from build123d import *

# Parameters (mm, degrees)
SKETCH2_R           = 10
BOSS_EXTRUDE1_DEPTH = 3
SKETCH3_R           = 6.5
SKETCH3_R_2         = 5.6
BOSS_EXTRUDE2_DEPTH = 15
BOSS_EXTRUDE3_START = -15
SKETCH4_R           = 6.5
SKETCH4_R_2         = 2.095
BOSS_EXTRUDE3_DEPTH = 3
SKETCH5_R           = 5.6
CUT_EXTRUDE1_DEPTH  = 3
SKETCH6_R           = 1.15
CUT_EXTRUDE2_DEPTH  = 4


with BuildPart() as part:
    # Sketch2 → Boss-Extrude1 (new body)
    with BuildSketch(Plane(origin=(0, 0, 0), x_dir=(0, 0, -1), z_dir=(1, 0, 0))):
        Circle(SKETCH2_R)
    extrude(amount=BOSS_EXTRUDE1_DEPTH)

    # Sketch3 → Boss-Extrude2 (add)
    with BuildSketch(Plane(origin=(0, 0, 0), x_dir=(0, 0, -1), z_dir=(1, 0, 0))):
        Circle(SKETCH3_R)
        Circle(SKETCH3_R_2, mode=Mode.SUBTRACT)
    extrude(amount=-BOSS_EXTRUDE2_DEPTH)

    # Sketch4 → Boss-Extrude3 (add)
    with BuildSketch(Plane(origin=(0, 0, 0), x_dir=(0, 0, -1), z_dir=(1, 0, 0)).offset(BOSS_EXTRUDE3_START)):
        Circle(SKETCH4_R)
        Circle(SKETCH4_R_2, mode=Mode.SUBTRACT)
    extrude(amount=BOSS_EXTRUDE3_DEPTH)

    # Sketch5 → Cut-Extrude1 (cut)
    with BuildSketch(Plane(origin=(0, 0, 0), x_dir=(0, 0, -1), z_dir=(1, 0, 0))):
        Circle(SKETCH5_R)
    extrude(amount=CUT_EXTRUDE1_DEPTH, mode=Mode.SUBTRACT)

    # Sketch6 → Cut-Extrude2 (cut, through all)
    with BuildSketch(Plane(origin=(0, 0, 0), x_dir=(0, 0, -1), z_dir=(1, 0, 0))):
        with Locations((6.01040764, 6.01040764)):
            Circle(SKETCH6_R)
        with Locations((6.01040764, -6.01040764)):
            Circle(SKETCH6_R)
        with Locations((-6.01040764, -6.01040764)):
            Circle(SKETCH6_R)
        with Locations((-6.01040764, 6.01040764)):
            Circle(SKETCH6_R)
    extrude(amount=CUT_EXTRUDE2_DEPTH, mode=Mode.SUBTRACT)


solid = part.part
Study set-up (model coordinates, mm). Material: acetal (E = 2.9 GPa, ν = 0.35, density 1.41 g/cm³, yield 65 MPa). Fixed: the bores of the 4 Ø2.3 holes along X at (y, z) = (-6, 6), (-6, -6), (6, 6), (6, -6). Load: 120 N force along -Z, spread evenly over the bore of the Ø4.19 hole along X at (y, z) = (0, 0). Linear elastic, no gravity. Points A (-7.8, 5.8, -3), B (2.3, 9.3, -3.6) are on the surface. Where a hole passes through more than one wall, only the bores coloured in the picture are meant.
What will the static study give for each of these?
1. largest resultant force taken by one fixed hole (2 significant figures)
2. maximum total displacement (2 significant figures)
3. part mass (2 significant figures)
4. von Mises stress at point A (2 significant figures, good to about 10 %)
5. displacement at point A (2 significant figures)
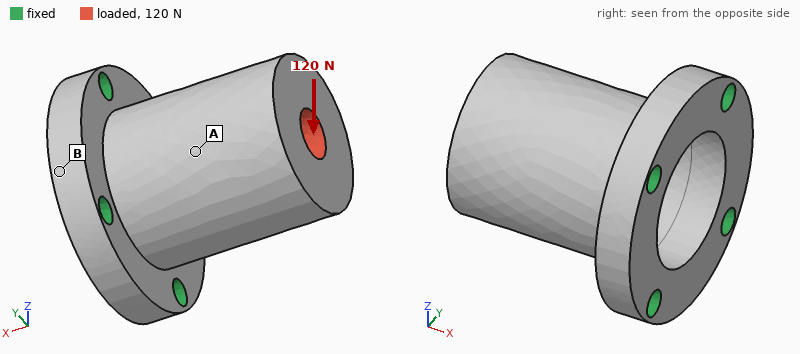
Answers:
87 N
0.21 mm
1.9 g
11 MPa
0.11 mm
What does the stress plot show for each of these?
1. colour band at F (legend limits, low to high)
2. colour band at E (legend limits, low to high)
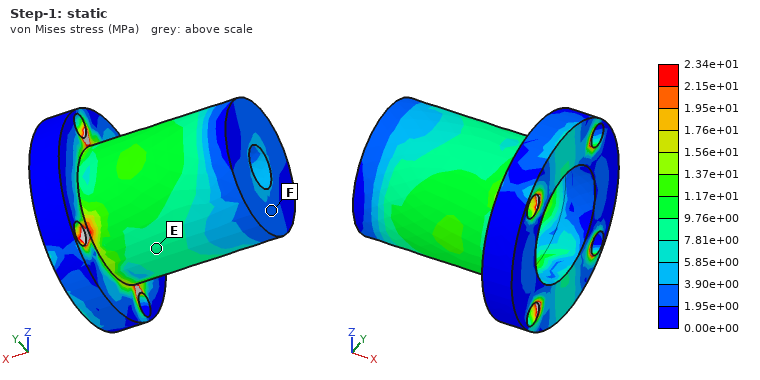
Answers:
1.95e+00 to 3.90e+00 MPa
7.81e+00 to 9.76e+00 MPa
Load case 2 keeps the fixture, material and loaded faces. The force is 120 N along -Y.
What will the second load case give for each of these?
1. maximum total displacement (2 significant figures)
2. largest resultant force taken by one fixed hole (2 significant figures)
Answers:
0.21 mm
87 N
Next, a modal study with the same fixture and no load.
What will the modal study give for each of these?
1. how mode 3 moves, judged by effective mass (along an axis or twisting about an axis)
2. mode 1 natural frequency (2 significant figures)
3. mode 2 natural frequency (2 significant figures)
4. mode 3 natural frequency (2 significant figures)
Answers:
twisting about X
4800 Hz
4900 Hz
11 kHz
